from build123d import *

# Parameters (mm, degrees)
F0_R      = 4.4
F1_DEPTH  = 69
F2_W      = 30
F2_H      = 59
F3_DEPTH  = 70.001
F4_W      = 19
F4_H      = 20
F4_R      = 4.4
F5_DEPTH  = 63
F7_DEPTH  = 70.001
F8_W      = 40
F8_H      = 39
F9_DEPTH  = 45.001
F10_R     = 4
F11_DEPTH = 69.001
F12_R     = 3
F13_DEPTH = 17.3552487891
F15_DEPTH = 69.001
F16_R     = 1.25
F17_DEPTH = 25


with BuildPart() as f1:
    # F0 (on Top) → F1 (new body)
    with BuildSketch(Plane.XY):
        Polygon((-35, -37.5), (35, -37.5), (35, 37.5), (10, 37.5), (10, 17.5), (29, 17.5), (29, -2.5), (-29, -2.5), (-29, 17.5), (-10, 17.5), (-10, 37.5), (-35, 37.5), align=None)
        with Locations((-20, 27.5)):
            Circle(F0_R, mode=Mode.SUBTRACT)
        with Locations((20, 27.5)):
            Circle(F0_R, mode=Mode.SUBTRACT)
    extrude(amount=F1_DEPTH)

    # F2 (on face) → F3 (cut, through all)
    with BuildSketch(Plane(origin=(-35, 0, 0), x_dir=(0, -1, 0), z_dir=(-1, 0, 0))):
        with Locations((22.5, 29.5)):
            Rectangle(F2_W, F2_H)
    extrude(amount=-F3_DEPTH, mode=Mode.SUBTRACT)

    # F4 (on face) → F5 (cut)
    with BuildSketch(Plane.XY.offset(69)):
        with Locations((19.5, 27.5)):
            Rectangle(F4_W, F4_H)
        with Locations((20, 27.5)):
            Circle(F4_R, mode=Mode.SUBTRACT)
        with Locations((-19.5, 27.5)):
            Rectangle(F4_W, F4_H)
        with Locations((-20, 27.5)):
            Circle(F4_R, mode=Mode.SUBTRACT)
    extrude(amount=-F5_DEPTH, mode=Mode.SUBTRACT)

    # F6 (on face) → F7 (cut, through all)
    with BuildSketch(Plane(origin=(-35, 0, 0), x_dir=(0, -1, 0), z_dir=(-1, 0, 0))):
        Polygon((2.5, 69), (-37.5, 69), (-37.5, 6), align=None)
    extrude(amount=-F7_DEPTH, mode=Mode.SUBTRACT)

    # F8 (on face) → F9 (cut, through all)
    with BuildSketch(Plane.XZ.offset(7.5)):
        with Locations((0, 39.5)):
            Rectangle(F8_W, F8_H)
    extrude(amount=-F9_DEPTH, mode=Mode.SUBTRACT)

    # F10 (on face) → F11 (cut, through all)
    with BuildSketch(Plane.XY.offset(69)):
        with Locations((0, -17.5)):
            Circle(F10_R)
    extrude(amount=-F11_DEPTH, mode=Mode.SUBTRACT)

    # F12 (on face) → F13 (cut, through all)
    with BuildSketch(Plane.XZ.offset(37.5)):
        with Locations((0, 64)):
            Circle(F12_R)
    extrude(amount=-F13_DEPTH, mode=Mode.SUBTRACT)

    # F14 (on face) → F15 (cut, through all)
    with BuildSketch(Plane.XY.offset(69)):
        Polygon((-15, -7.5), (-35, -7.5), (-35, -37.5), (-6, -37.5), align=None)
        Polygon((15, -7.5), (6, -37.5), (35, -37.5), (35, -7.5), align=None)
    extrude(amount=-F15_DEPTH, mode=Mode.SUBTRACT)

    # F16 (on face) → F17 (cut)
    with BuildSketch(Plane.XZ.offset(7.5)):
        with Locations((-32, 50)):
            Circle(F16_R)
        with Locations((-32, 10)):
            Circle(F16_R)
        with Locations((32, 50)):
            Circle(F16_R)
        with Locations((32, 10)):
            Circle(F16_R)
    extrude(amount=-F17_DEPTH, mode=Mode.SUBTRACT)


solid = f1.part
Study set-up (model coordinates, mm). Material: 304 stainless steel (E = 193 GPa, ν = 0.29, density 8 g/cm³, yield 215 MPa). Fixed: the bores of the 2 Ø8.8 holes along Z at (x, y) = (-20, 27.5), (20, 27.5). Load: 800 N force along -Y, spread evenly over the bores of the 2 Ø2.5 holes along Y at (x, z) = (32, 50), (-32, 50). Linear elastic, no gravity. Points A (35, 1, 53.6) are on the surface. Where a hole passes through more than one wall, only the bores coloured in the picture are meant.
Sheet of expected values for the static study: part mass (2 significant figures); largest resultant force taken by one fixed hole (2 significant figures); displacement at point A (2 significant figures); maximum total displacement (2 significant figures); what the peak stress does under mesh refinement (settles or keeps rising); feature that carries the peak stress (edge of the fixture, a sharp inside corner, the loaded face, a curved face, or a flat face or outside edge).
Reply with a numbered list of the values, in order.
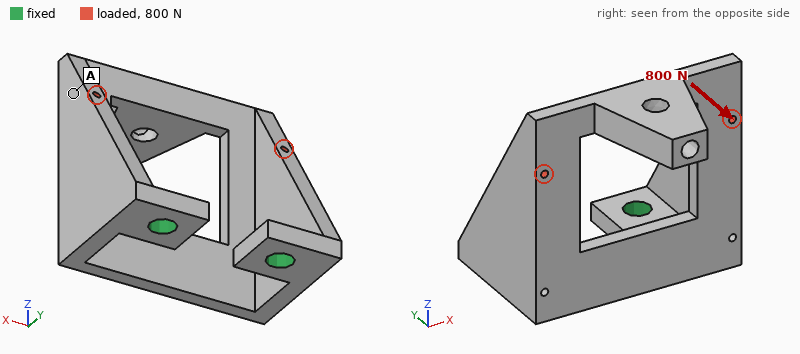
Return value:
1. 340 g
2. 400 N
3. 0.084 mm
4. 0.14 mm
5. keeps rising
6. edge of the fixture
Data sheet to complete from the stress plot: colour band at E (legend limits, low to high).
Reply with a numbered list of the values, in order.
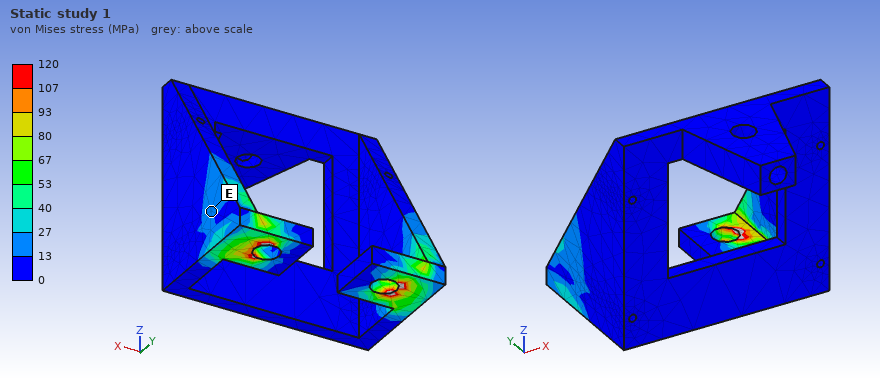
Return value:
1. 13 to 27 MPa
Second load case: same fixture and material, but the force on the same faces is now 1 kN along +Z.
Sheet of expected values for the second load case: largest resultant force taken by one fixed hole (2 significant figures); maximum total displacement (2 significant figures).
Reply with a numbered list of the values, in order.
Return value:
1. 500 N
2. 92 µm
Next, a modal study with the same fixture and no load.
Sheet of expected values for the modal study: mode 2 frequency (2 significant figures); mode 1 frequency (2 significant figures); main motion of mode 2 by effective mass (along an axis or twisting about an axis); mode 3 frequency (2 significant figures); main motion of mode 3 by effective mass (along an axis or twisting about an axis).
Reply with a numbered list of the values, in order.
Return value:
1. 1200 Hz
2. 930 Hz
3. along X
4. 2100 Hz
5. along X
